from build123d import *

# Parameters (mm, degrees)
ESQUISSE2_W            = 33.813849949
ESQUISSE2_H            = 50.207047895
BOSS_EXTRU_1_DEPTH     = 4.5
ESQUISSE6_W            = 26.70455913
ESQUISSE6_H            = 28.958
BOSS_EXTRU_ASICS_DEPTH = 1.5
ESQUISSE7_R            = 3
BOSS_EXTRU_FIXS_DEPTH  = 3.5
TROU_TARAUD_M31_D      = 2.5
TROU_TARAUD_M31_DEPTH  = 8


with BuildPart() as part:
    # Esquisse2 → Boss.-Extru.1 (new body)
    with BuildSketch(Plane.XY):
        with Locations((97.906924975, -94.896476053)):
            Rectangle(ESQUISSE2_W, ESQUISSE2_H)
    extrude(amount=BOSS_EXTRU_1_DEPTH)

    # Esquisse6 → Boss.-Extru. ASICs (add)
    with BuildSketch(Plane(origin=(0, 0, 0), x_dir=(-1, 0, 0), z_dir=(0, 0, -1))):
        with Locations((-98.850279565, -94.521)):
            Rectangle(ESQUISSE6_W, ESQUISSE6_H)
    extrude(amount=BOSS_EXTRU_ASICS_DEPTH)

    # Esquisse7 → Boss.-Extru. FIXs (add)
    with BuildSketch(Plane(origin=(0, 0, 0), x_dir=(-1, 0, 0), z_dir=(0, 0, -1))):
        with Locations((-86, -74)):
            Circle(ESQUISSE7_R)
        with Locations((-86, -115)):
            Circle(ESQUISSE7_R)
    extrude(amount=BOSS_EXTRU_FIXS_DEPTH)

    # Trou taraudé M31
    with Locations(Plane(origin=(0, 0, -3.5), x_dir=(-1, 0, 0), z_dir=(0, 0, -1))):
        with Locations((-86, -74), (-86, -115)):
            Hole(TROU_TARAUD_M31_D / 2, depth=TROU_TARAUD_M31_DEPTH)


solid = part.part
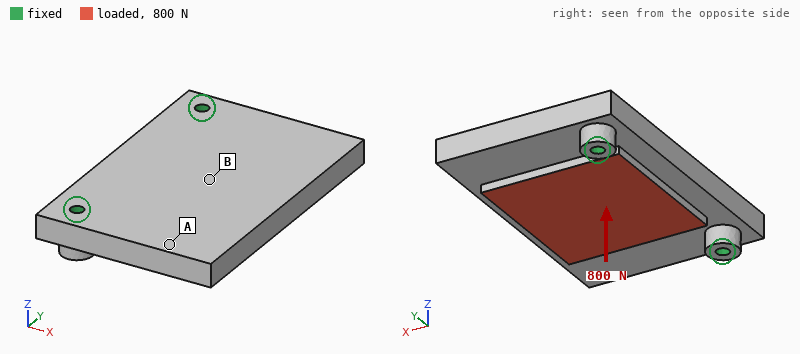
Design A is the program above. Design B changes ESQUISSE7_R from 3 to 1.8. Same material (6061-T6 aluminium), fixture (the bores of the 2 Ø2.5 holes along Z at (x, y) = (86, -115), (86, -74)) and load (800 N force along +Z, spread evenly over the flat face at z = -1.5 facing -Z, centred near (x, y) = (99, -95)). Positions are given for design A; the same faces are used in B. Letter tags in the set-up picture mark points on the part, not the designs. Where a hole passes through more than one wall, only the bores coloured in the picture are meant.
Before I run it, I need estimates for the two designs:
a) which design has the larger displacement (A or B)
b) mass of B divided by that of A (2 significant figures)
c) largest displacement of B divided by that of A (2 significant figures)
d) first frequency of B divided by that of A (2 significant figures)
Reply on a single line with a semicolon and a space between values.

B; 0.99; 1.1; 0.94
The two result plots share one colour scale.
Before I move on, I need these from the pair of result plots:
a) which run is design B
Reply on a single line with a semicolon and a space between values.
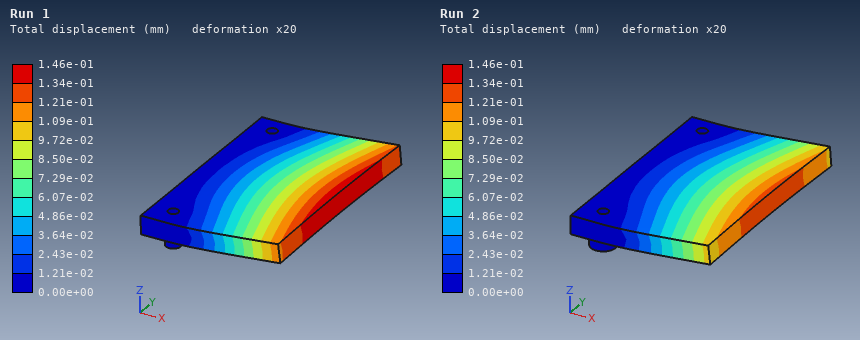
Run 1
